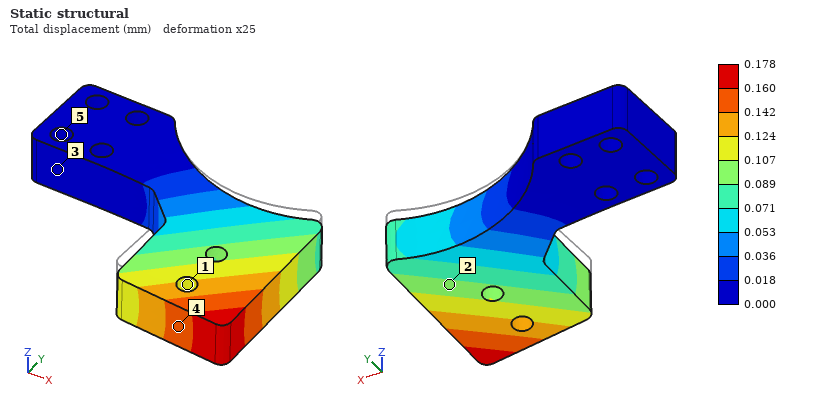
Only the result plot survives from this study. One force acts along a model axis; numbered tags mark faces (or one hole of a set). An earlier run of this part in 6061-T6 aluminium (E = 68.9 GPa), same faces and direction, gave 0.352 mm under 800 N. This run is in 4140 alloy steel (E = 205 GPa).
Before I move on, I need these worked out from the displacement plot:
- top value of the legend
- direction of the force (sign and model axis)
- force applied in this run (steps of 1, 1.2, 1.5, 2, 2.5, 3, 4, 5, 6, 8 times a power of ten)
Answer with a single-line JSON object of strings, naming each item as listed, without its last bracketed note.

{"top value of the legend": "0.178 mm", "direction of the force": "-Z", "force applied in this run": "1.2 kN"}
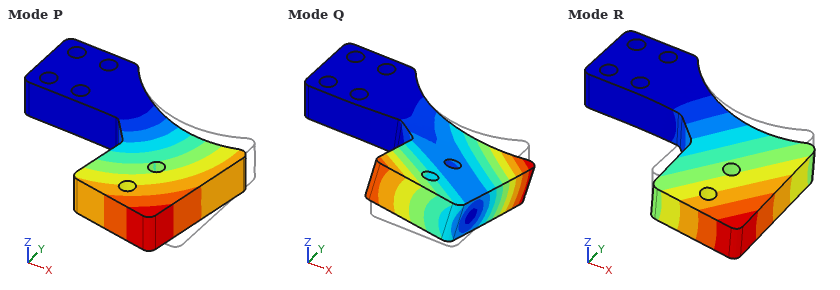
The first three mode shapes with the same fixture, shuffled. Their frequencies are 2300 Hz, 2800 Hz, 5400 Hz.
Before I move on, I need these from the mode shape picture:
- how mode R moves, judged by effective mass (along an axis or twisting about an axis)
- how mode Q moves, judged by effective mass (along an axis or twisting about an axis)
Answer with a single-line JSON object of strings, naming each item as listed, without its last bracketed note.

{"how mode R moves, judged by effective mass": "along Z", "how mode Q moves, judged by effective mass": "twisting about X"}
